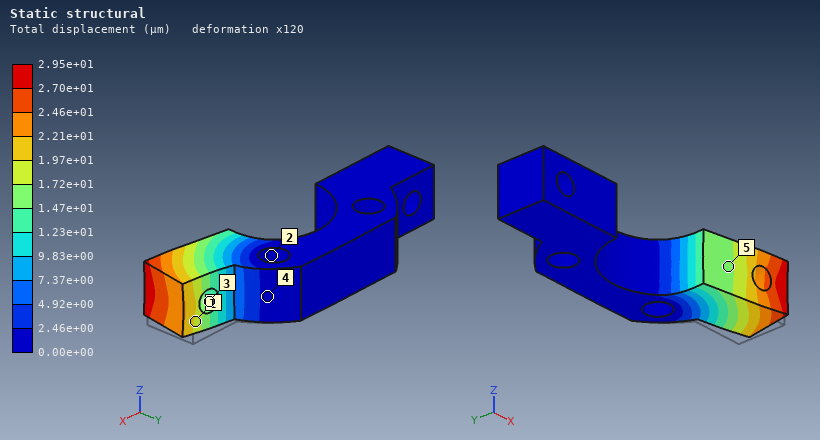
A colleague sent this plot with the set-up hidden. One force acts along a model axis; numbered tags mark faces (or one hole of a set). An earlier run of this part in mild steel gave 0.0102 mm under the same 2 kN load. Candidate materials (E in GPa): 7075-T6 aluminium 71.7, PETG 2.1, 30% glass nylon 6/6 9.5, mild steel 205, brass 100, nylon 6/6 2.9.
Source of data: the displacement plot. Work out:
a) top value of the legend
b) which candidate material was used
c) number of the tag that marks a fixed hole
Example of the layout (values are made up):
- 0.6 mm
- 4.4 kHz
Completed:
- 2.95e+01 µm
- 7075-T6 aluminium
- 2
